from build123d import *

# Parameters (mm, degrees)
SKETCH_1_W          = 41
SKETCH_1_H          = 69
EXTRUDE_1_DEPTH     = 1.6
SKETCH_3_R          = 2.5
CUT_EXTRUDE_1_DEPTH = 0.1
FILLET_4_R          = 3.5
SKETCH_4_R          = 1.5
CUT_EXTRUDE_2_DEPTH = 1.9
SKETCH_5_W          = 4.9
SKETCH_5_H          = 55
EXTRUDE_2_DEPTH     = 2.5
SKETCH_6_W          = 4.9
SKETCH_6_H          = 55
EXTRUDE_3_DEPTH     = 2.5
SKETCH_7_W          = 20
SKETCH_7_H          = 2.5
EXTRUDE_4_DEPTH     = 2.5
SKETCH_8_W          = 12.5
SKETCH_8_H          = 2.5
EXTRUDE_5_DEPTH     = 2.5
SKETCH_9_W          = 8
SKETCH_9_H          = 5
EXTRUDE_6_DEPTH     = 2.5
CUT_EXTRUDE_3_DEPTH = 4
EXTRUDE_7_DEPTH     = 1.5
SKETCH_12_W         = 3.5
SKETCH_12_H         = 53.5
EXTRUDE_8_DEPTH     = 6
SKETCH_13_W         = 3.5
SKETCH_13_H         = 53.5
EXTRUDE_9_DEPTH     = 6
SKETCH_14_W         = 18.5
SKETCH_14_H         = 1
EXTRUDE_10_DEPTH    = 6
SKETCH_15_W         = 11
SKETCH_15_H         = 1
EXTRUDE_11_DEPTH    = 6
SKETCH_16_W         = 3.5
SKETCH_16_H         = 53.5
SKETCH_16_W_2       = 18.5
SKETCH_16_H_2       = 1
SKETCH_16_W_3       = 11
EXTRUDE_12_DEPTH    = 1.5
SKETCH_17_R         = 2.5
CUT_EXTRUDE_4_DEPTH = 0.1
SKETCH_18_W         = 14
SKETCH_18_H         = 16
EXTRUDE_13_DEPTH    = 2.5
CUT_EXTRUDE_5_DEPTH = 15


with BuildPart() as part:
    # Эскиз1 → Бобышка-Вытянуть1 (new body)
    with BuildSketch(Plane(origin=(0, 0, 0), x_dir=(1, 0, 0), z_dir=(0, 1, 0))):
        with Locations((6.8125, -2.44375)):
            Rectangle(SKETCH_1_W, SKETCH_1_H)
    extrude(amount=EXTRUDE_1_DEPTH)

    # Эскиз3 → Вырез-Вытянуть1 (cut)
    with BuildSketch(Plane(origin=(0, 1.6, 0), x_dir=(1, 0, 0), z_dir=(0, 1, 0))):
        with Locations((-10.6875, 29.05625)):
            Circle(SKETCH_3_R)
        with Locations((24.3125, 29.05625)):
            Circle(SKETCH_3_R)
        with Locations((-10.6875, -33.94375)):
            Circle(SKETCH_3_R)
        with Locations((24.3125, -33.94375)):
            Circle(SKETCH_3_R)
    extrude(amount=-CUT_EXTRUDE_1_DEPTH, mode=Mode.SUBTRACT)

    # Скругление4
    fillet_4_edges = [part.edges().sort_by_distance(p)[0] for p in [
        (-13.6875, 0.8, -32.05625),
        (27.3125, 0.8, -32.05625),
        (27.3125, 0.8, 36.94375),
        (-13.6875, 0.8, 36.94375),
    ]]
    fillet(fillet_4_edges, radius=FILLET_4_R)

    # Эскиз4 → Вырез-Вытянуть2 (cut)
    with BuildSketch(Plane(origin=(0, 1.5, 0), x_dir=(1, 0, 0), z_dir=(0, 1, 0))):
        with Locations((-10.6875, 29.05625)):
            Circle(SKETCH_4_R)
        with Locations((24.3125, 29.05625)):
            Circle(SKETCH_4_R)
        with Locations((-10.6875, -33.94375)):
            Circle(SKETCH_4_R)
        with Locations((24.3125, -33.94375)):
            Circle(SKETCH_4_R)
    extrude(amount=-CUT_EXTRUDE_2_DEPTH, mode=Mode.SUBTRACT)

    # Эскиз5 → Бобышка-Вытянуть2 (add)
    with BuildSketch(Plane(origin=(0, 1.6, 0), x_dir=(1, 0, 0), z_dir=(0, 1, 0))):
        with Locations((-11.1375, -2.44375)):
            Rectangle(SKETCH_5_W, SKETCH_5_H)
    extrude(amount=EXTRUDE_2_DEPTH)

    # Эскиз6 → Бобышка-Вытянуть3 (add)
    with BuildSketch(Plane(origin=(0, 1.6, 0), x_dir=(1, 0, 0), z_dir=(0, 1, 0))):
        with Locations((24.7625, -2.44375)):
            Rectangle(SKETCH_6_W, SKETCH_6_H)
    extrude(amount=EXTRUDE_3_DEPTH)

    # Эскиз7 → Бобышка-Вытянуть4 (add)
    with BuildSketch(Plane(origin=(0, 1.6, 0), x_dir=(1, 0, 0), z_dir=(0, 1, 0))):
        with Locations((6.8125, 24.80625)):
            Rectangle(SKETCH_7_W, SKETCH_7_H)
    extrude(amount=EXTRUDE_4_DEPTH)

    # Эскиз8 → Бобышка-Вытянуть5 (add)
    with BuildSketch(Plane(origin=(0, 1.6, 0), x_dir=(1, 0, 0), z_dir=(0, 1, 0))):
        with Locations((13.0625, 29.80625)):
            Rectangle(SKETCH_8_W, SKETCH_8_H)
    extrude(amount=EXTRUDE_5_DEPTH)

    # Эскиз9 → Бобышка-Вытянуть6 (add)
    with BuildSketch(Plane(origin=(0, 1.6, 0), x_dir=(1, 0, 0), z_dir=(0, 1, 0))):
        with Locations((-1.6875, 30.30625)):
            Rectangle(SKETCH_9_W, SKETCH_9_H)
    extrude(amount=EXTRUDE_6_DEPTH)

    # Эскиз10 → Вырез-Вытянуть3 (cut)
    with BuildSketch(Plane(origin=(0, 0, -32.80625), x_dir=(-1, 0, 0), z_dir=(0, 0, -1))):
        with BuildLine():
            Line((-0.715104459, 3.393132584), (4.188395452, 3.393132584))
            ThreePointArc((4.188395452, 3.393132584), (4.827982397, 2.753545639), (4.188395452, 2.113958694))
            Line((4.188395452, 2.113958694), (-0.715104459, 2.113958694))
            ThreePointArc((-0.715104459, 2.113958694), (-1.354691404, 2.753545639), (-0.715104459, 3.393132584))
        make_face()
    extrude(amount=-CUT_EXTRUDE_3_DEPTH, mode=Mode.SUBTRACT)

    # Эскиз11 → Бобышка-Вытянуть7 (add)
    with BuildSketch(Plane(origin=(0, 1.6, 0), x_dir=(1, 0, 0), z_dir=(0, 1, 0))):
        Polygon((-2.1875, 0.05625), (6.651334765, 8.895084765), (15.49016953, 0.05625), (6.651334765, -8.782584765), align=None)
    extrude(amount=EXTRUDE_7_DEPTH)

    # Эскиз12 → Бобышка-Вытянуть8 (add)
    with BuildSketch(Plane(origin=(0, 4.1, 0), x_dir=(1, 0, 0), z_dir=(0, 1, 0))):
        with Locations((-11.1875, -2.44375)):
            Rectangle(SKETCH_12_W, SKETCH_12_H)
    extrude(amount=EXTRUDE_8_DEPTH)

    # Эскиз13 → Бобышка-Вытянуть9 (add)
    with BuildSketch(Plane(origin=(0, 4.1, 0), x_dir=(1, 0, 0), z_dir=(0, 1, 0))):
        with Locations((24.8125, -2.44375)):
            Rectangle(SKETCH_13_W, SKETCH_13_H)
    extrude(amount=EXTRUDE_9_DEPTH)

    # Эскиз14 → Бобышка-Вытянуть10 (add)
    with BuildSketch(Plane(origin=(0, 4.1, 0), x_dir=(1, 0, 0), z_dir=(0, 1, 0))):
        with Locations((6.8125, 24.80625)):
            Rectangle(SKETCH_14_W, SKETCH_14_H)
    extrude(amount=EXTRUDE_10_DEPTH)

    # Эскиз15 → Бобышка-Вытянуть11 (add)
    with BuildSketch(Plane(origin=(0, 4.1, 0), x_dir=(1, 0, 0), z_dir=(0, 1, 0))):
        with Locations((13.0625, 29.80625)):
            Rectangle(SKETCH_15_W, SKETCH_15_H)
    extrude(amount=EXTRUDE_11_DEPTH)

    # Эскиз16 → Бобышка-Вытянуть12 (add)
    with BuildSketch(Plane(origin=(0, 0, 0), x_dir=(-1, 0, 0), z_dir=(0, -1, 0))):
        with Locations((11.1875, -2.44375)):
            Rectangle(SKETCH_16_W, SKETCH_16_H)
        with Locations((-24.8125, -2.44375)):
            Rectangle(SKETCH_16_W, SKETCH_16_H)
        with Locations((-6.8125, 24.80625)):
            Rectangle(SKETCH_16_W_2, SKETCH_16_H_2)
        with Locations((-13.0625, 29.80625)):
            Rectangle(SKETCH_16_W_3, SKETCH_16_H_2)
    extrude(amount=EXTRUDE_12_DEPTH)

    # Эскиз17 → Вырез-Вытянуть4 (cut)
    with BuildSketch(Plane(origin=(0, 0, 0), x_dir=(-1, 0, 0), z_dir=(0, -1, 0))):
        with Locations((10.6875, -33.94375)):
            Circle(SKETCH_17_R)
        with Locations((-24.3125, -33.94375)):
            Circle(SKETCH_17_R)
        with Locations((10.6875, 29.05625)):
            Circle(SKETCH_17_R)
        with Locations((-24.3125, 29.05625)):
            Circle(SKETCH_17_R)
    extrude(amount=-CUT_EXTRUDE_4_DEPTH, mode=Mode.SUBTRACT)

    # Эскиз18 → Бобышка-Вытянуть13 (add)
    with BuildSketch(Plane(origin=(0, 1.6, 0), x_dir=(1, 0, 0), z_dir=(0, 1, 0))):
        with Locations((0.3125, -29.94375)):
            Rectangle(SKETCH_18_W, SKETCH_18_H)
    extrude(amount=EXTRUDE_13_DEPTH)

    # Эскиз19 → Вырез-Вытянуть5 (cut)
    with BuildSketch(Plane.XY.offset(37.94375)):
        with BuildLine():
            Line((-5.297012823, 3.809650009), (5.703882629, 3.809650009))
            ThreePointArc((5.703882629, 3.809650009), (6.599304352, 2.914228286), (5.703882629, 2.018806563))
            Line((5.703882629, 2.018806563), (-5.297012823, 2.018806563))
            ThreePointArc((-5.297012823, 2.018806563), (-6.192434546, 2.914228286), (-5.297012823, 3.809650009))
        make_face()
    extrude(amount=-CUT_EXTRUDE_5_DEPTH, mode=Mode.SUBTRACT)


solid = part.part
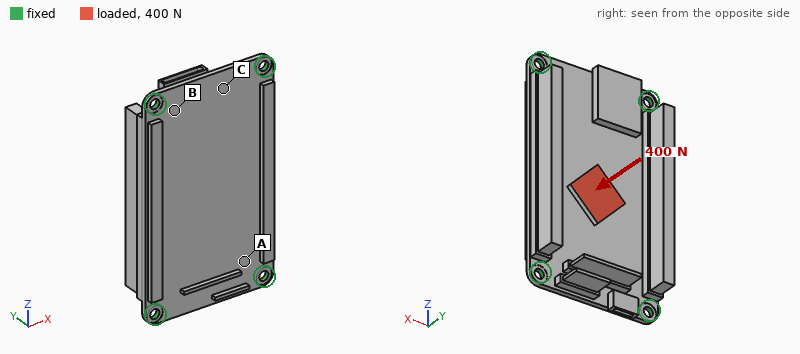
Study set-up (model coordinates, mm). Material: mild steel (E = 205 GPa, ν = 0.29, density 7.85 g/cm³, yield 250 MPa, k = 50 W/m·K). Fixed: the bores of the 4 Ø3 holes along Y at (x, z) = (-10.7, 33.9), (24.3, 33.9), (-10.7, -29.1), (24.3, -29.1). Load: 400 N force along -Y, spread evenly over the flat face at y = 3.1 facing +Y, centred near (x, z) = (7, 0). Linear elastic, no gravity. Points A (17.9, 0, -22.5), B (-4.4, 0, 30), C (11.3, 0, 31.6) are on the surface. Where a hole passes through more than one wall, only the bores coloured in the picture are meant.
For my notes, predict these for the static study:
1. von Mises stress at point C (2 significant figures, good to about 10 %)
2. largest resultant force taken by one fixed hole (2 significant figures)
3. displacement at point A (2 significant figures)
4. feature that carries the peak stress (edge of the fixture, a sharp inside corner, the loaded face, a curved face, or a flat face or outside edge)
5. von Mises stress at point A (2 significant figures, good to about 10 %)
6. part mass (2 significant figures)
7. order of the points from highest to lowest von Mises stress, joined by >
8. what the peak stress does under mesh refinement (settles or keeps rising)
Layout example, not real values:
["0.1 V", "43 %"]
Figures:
["17 MPa", "180 N", "9.8 µm", "edge of the fixture", "30 MPa", "75 g", "A > C > B", "keeps rising"]
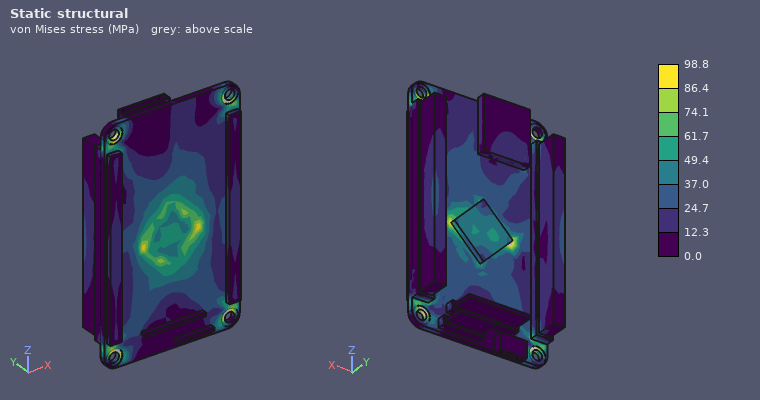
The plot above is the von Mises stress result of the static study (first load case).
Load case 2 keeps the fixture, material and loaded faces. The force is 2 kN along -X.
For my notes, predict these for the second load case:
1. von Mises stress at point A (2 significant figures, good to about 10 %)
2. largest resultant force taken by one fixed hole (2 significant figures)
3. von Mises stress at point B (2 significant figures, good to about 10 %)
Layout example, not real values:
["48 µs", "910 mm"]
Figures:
["37 MPa", "720 N", "27 MPa"]
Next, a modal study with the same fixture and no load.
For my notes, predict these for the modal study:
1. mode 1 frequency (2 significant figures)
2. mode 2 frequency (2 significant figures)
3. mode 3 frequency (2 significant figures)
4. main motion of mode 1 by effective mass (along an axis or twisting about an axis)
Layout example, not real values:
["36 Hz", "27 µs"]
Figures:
["4200 Hz", "6600 Hz", "6700 Hz", "along Y"]
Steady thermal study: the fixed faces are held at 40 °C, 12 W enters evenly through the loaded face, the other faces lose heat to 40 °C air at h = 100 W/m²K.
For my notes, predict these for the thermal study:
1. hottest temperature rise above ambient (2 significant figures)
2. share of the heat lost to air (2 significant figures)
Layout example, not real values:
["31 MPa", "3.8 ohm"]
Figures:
["38 K", "73 %"]
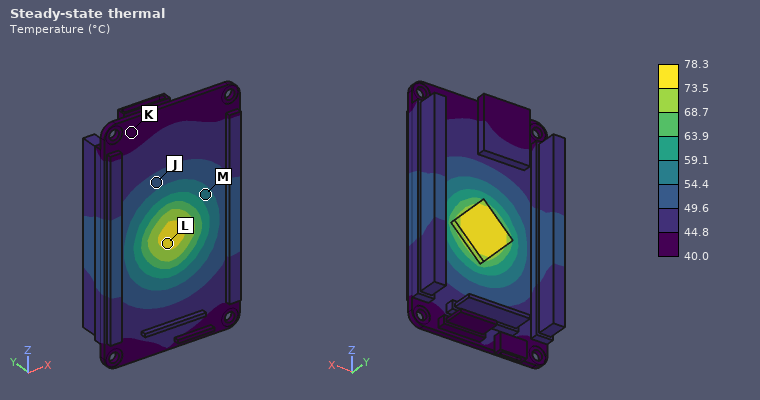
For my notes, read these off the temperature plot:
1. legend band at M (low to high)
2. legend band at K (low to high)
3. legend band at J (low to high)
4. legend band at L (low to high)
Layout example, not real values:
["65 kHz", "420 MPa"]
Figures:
["54.4 to 59.1 °C", "40.0 to 44.8 °C", "49.6 to 54.4 °C", "73.5 to 78.3 °C"]
